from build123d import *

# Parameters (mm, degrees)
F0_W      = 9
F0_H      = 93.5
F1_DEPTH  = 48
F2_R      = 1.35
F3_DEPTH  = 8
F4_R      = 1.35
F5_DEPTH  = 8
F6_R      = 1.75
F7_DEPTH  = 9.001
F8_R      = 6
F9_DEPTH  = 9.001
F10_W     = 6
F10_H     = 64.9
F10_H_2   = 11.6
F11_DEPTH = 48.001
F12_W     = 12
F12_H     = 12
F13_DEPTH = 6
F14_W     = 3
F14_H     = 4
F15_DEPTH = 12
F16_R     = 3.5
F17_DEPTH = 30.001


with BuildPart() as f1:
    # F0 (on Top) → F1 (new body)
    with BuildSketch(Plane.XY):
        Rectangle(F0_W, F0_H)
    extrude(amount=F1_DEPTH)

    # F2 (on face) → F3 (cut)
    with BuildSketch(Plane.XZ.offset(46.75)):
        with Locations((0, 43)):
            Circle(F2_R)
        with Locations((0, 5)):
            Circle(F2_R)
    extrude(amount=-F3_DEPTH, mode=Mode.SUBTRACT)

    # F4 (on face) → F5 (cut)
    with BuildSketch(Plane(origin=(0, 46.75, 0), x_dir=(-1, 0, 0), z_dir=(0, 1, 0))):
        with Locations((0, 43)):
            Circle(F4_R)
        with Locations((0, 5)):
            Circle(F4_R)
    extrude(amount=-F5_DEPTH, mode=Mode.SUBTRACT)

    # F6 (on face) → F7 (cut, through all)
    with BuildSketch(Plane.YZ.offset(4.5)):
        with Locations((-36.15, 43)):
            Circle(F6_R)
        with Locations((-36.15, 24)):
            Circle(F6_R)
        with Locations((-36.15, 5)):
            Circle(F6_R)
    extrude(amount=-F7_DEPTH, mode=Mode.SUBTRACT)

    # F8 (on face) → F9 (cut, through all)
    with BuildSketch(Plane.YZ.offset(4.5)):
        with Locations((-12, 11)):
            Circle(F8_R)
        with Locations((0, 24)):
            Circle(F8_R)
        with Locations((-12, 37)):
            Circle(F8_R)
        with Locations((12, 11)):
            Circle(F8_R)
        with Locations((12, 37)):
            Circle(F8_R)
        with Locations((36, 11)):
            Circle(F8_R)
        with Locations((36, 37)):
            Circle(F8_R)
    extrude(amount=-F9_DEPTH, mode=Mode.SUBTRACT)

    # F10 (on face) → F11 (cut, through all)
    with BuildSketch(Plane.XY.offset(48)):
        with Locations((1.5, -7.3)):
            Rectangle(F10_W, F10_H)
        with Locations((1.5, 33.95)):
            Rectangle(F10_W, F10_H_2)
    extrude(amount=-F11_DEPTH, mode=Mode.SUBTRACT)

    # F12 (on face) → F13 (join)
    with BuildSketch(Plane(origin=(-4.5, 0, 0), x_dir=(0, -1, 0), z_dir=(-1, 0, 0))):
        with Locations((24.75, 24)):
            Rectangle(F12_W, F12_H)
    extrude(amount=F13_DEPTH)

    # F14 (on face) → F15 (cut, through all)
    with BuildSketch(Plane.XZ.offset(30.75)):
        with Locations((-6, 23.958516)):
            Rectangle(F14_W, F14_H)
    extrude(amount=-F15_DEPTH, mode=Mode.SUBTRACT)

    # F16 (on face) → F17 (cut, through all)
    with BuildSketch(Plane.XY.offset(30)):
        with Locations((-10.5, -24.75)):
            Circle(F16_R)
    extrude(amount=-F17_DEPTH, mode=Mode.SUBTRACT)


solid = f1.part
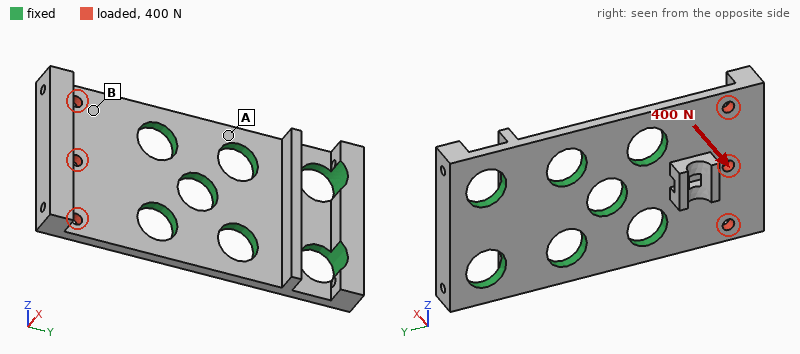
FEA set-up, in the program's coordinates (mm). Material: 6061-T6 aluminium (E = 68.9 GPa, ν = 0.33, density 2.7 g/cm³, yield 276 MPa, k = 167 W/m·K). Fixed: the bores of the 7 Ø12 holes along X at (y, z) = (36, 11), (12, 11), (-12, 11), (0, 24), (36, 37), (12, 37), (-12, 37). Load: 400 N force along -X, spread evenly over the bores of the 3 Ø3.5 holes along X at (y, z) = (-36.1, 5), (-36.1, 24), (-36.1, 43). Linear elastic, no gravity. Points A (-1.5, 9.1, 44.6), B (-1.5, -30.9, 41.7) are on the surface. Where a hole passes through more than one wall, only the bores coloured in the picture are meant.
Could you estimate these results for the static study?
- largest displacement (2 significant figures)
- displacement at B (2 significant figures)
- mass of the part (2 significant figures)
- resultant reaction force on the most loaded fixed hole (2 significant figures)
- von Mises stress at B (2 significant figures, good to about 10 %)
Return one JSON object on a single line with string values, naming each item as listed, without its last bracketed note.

{"largest displacement": "0.20 mm", "displacement at B": "0.067 mm", "mass of the part": "43 g", "resultant reaction force on the most loaded fixed hole": "230 N", "von Mises stress at B": "21 MPa"}
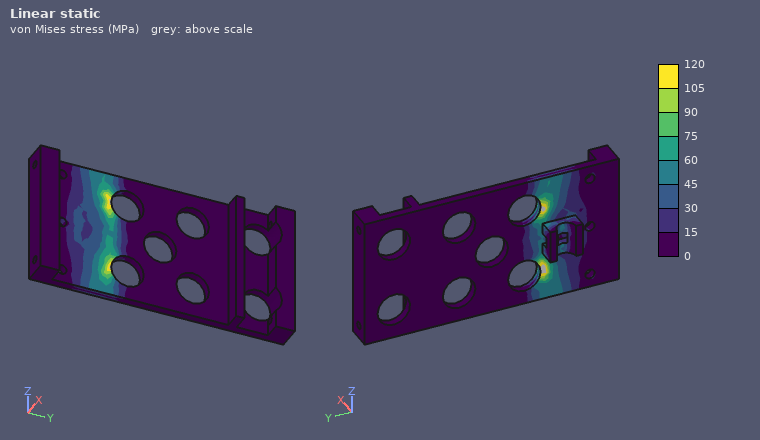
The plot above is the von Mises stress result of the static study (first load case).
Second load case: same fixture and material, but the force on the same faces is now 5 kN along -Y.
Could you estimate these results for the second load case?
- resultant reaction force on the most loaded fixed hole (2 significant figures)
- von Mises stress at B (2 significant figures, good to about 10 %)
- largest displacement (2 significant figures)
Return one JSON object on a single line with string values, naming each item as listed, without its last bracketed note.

{"resultant reaction force on the most loaded fixed hole": "2.3 kN", "von Mises stress at B": "47 MPa", "largest displacement": "19 µm"}
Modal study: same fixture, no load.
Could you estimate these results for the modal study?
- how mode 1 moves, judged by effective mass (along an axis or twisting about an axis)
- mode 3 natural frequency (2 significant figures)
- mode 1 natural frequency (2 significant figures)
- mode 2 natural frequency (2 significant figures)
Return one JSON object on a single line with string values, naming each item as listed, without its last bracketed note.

{"how mode 1 moves, judged by effective mass": "along X", "mode 3 natural frequency": "11 kHz", "mode 1 natural frequency": "2000 Hz", "mode 2 natural frequency": "4100 Hz"}
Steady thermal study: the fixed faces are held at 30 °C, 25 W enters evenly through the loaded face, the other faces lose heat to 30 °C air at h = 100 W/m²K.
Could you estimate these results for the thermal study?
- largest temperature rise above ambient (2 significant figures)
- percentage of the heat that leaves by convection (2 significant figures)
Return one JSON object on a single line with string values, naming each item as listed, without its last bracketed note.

{"largest temperature rise above ambient": "20 K", "percentage of the heat that leaves by convection": "21 %"}
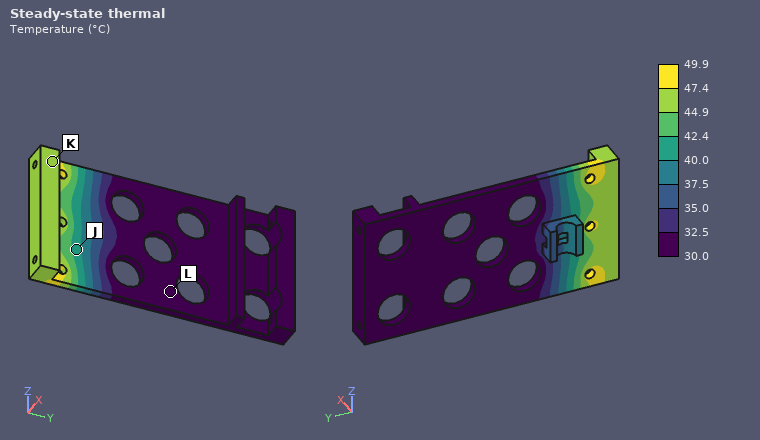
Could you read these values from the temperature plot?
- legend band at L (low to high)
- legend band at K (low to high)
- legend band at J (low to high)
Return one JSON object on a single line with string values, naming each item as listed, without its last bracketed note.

{"legend band at L": "30.0 to 32.5 °C", "legend band at K": "44.9 to 47.4 °C", "legend band at J": "40.0 to 42.4 °C"}
